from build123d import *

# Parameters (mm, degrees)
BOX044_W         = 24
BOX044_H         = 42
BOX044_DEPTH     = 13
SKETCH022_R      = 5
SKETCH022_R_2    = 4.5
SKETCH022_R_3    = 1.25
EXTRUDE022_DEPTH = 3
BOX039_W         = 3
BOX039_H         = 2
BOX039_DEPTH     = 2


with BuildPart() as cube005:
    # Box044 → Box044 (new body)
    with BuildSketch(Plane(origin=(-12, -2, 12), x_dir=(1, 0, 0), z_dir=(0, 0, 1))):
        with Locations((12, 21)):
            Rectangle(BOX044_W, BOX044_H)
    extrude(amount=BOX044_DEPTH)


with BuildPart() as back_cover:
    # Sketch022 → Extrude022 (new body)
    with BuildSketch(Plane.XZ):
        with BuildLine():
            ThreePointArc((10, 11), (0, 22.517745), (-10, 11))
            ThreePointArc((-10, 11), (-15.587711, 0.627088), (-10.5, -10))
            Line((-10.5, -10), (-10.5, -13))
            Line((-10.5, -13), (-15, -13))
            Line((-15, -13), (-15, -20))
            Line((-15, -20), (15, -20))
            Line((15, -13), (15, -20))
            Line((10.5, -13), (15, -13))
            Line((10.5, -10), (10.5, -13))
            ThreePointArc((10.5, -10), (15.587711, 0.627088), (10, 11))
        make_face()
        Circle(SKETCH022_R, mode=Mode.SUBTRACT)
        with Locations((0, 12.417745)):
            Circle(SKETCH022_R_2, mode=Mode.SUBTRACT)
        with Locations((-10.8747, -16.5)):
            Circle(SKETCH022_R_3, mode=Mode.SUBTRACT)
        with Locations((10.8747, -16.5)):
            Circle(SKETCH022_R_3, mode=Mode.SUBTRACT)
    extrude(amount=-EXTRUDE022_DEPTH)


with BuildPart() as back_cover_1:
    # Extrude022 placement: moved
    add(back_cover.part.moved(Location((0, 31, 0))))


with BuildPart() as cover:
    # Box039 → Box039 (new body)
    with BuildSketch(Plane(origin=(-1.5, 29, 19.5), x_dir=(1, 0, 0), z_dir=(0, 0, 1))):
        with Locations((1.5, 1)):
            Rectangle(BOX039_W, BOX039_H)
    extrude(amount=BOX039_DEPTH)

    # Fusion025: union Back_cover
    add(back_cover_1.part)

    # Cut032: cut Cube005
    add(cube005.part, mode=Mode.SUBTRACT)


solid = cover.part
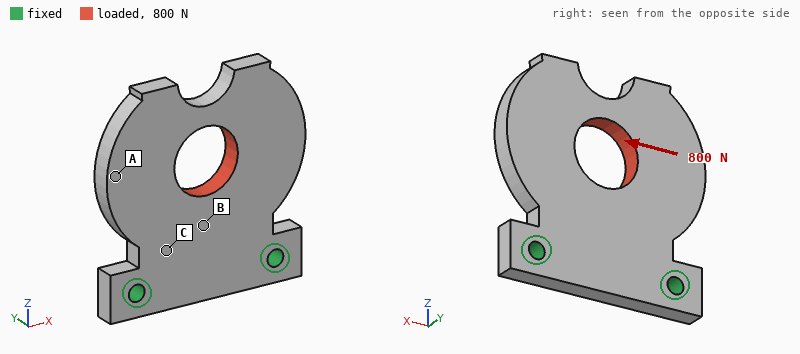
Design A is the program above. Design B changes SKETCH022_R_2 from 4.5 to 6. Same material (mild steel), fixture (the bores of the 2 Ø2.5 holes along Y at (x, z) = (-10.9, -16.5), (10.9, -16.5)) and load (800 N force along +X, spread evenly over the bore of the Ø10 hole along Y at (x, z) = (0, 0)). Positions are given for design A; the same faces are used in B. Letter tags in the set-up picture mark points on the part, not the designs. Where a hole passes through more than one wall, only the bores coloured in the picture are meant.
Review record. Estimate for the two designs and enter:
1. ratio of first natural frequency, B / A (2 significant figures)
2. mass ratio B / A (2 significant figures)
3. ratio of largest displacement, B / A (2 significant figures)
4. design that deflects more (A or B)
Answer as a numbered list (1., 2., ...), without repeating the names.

1. 1.1
2. 0.97
3. 1.1
4. B
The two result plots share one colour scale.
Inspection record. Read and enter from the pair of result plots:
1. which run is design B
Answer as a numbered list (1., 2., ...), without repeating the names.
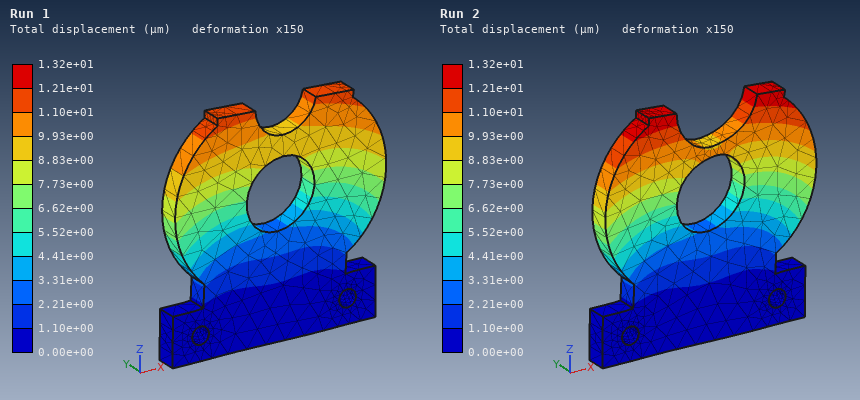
1. Run 2
